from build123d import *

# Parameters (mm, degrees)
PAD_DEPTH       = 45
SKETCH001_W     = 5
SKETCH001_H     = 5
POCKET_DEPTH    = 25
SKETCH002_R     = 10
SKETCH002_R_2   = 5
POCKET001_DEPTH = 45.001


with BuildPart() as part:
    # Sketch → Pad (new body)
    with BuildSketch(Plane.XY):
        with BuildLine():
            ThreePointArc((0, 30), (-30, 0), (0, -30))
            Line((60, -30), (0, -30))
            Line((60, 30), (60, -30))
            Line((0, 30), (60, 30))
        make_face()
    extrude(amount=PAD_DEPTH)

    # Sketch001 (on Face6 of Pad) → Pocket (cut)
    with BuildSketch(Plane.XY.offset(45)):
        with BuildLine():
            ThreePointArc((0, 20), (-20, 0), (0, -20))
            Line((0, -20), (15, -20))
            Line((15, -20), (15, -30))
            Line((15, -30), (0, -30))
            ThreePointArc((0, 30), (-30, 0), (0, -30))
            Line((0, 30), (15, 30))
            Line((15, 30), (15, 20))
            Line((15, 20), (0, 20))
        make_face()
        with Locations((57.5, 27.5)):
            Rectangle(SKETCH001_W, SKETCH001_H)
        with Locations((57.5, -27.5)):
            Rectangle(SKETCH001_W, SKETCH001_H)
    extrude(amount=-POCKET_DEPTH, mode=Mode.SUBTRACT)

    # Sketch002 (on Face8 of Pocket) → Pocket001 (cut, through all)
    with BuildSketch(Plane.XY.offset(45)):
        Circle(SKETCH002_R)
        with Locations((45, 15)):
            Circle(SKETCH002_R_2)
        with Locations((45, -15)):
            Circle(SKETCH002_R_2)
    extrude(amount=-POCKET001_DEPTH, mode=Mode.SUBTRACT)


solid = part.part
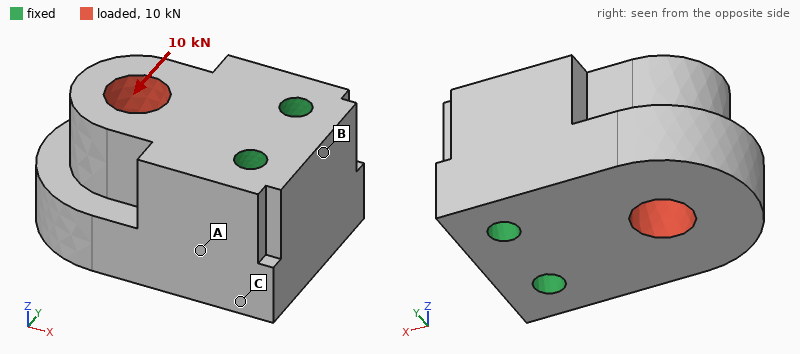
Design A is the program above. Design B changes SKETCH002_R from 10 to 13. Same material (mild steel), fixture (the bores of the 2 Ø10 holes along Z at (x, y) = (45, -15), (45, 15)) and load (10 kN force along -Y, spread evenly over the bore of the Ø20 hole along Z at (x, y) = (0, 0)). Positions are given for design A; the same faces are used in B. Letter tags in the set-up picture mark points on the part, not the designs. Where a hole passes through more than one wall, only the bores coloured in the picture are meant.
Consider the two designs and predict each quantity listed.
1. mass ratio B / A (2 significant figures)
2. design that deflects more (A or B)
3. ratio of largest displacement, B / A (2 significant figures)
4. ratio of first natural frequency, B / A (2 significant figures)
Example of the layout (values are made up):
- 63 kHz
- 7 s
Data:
- 0.94
- B
- 1.4
- 1.00
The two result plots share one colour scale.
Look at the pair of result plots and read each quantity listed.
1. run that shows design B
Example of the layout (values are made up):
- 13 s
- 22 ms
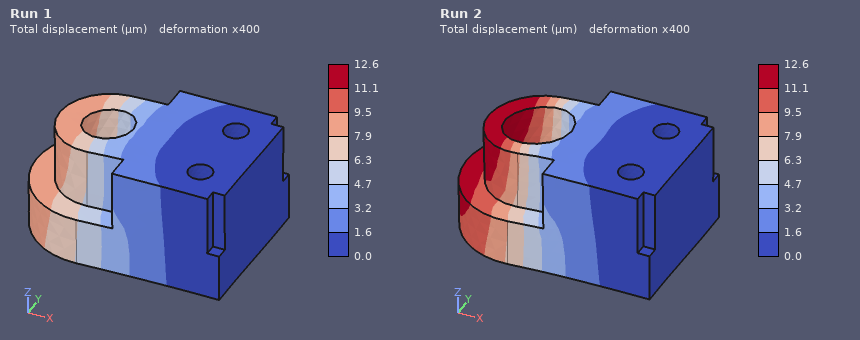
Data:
- Run 2
